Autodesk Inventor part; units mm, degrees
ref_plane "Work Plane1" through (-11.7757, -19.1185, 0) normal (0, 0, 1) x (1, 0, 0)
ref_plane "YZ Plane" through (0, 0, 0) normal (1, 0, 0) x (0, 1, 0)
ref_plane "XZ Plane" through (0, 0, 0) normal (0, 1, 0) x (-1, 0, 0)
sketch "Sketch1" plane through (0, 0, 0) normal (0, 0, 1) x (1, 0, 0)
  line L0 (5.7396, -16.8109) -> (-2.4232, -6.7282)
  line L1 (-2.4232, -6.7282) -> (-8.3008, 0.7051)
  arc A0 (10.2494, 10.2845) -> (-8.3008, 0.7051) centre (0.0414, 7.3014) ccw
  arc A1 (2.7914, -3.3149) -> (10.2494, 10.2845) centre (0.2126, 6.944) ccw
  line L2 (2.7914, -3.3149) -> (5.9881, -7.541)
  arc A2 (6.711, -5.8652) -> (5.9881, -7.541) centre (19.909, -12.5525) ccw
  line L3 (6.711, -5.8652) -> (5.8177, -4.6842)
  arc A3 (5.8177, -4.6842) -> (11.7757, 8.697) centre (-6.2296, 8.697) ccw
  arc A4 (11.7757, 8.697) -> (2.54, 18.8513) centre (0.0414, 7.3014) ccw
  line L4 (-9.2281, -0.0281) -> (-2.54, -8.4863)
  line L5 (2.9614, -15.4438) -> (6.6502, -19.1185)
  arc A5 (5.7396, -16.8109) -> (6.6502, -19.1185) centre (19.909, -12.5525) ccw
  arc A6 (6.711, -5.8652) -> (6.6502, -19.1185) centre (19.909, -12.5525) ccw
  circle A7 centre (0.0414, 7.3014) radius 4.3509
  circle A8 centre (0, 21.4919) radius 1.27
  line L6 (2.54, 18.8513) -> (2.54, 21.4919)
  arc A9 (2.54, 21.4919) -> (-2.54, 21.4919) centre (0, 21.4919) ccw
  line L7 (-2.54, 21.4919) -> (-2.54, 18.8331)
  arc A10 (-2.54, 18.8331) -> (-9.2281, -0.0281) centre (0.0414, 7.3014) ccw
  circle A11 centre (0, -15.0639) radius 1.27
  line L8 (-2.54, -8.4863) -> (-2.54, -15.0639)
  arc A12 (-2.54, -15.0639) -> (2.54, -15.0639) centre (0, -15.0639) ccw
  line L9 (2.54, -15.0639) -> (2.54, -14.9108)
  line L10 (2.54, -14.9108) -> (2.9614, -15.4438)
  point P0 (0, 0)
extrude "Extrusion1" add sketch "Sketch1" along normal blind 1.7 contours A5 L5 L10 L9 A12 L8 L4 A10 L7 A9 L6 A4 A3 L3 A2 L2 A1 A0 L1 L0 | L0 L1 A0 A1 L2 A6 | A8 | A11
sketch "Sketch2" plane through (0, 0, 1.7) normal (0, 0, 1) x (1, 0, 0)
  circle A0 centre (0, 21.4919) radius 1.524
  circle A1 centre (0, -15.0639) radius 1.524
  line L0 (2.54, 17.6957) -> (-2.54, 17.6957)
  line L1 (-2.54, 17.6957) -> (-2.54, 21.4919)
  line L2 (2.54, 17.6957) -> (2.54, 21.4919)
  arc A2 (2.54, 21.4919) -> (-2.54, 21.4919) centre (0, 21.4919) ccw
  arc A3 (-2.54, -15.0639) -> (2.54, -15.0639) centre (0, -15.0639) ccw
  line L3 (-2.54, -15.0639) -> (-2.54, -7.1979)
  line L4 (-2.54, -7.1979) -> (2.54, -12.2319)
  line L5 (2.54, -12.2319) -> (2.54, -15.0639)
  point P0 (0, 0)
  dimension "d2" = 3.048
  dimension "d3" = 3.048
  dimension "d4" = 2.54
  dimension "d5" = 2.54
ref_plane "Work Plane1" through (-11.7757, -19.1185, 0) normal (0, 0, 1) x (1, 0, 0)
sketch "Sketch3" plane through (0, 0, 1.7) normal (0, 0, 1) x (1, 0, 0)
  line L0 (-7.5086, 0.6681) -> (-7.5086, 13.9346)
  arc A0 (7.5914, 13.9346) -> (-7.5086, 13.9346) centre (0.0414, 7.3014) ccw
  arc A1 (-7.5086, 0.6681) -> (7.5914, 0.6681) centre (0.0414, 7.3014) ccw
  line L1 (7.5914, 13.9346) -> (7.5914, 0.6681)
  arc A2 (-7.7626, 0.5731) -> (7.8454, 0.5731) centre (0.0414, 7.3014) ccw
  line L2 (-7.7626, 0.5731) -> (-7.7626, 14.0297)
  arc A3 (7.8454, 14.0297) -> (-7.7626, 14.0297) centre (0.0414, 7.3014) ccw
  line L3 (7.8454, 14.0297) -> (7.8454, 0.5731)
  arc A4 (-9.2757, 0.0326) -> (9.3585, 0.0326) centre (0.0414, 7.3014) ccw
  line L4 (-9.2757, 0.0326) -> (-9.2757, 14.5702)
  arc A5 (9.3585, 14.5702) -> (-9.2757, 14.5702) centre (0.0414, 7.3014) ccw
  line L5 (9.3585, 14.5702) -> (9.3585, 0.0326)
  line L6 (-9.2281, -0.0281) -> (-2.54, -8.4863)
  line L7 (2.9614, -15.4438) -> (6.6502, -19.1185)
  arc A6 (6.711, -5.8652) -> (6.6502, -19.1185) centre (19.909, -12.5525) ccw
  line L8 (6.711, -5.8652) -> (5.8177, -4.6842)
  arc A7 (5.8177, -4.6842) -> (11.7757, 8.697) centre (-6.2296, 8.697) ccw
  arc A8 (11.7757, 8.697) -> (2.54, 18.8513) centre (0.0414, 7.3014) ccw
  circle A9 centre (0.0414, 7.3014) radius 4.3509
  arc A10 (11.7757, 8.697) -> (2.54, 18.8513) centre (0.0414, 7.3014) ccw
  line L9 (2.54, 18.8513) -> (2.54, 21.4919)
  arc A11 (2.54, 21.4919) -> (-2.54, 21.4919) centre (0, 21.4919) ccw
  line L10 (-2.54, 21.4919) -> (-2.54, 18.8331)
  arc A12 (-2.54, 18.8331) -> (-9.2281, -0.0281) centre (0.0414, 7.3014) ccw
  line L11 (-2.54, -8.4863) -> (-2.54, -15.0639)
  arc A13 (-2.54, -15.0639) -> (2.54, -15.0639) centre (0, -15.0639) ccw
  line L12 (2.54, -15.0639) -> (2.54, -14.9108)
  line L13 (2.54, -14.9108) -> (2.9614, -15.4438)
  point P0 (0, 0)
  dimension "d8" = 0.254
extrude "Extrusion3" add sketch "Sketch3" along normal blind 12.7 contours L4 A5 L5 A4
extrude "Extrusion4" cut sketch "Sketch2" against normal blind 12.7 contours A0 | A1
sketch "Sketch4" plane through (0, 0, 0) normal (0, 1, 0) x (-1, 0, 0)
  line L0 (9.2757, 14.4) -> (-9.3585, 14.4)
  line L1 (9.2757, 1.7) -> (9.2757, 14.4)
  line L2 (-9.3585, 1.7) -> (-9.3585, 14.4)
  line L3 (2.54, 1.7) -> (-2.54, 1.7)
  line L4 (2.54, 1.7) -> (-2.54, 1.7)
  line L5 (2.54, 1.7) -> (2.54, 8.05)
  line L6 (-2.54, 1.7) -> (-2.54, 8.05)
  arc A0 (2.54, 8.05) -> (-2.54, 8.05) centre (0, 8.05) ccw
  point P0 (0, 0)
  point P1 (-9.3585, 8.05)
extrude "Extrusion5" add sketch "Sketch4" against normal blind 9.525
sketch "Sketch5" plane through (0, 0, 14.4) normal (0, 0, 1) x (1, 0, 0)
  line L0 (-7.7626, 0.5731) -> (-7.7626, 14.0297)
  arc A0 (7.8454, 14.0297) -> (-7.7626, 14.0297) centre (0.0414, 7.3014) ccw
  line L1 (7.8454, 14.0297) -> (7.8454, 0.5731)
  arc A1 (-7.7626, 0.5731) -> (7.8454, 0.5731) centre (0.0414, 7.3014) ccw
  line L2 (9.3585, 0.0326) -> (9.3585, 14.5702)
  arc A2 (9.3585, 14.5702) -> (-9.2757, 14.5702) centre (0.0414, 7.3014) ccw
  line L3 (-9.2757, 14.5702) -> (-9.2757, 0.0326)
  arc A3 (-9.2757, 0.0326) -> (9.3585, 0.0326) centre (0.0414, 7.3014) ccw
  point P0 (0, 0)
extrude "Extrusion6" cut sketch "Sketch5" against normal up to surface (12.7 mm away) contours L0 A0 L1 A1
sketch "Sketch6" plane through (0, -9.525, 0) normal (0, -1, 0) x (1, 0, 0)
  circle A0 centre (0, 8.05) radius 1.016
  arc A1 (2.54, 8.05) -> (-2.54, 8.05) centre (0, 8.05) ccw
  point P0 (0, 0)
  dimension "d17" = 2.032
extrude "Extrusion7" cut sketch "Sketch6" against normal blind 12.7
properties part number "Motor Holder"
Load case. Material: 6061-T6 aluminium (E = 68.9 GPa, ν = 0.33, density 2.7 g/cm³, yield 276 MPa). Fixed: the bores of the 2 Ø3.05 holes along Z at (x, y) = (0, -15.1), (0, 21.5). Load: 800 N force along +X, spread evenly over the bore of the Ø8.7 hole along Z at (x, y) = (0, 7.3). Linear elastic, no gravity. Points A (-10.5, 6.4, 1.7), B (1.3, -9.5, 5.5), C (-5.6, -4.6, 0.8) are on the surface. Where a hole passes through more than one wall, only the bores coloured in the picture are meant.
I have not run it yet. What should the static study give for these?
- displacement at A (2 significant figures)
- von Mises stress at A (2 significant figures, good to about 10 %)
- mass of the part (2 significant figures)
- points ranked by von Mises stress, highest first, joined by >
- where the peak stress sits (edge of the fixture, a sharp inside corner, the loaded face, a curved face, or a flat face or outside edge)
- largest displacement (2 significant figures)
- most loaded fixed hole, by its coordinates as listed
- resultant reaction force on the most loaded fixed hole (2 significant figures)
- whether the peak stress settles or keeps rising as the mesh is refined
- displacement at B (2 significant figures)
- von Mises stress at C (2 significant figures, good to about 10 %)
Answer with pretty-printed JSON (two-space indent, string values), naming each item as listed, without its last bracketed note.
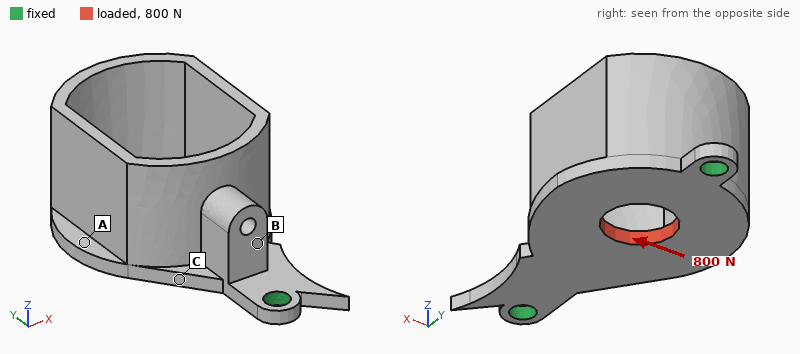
{
  "displacement at A": "17 µm",
  "von Mises stress at A": "18 MPa",
  "mass of the part": "6.3 g",
  "points ranked by von Mises stress, highest first, joined by >": "C > A > B",
  "where the peak stress sits": "edge of the fixture",
  "largest displacement": "21 µm",
  "most loaded fixed hole, by its coordinates as listed": "(0, 21.5)",
  "resultant reaction force on the most loaded fixed hole": "490 N",
  "whether the peak stress settles or keeps rising as the mesh is refined": "keeps rising",
  "displacement at B": "13 µm",
  "von Mises stress at C": "50 MPa"
}
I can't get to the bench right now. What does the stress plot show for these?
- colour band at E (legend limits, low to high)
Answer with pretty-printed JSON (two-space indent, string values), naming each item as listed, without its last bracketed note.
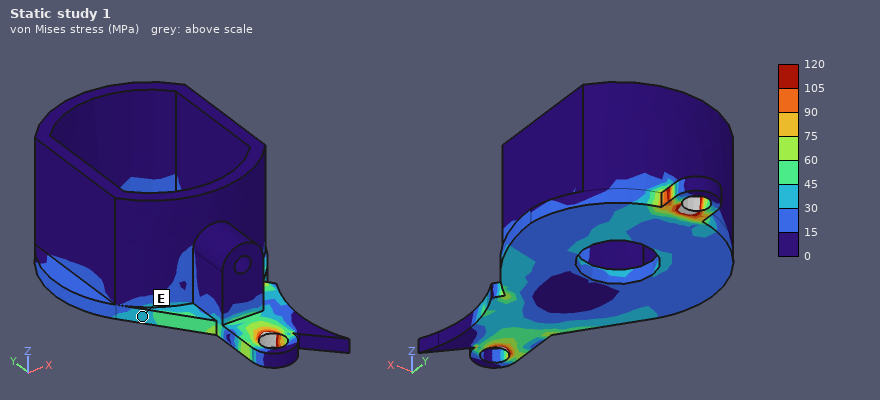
{
  "colour band at E": "30 to 45 MPa"
}
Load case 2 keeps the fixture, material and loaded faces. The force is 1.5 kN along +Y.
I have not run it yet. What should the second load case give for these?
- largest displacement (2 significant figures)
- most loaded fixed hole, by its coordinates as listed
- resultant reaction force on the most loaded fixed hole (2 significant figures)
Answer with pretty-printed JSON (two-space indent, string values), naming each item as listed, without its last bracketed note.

{
  "largest displacement": "13 µm",
  "most loaded fixed hole, by its coordinates as listed": "(0, 21.5)",
  "resultant reaction force on the most loaded fixed hole": "840 N"
}
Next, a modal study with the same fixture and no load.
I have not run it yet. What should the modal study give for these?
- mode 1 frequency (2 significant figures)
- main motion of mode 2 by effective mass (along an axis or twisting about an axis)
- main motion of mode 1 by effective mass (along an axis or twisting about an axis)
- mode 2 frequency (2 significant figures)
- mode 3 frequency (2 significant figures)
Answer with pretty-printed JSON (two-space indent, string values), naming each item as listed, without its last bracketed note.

{
  "mode 1 frequency": "3200 Hz",
  "main motion of mode 2 by effective mass": "along Z",
  "main motion of mode 1 by effective mass": "along X",
  "mode 2 frequency": "7600 Hz",
  "mode 3 frequency": "11 kHz"
}
